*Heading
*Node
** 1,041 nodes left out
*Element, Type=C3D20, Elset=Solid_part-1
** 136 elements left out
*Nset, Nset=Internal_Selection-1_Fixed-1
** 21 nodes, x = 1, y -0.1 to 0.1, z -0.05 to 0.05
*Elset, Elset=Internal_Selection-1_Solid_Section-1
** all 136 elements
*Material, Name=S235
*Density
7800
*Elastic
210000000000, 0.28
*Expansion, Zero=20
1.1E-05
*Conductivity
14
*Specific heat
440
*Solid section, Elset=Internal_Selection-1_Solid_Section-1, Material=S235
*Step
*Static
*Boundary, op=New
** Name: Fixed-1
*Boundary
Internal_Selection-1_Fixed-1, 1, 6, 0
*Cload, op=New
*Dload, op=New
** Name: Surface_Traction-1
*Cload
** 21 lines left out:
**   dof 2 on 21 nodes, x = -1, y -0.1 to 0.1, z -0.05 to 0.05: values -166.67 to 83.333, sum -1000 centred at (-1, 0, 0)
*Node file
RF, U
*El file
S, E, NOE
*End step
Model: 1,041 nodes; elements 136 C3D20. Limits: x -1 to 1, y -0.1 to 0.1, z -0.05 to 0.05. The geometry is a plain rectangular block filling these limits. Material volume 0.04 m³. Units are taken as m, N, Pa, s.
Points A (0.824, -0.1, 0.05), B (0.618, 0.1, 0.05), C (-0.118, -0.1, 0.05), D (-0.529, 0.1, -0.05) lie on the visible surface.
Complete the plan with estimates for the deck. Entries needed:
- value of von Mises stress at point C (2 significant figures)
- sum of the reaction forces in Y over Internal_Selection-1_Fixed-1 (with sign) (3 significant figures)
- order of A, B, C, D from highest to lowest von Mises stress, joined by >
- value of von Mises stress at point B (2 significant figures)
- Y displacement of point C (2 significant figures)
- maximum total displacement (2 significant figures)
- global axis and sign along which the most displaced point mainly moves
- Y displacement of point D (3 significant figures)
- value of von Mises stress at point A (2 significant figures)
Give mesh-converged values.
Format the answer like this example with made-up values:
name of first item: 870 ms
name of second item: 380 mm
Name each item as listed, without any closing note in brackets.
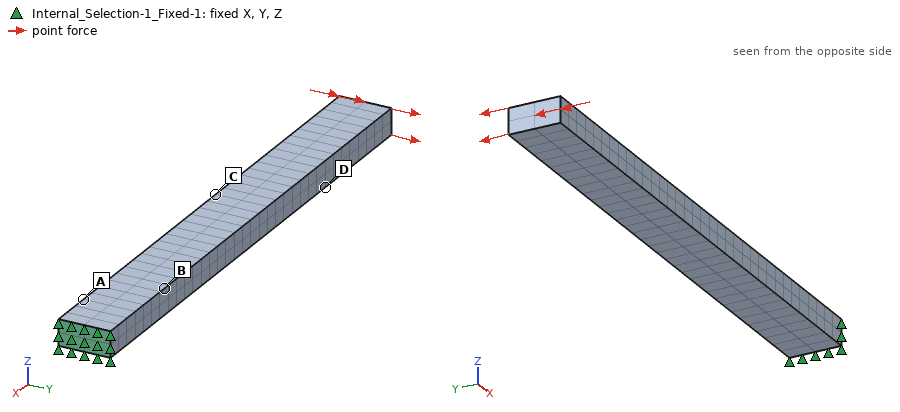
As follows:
value of von Mises stress at point C: 1.3e+06 Pa
sum of the reaction forces in Y over Internal_Selection-1_Fixed-1 (with sign): 1000 N
order of A, B, C, D from highest to lowest von Mises stress, joined by >: A > B > C > D
value of von Mises stress at point B: 2.4e+06 Pa
Y displacement of point C: -7.3e-05 m
maximum total displacement: 1.9e-04 m
global axis and sign along which the most displaced point mainly moves: -Y
Y displacement of point D: -1.25e-04 m
value of von Mises stress at point A: 2.7e+06 Pa
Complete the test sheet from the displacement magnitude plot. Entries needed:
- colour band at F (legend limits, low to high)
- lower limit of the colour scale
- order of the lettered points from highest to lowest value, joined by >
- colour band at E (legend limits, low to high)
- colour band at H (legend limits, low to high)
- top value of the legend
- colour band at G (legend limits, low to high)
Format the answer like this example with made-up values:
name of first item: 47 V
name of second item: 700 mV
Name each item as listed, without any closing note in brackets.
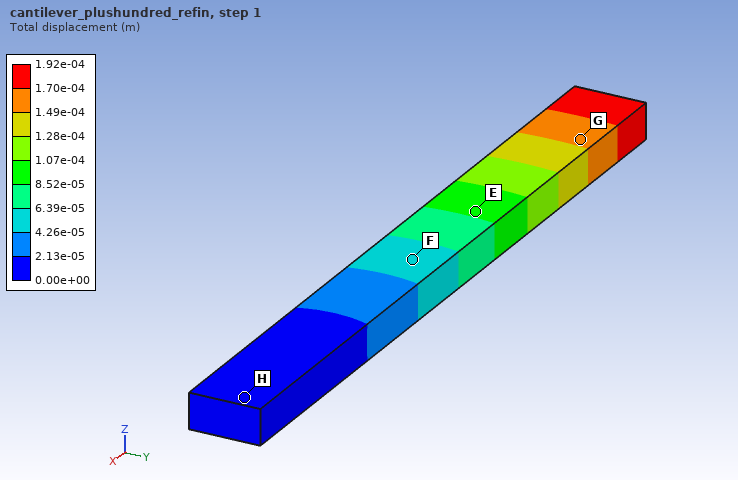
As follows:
colour band at F: 4.26e-05 to 6.39e-05 m
lower limit of the colour scale: 0.00e+00 m
order of the lettered points from highest to lowest value, joined by >: G > E > F > H
colour band at E: 8.52e-05 to 1.07e-04 m
colour band at H: 0.00e+00 to 2.13e-05 m
top value of the legend: 1.92e-04 m
colour band at G: 1.49e-04 to 1.70e-04 m
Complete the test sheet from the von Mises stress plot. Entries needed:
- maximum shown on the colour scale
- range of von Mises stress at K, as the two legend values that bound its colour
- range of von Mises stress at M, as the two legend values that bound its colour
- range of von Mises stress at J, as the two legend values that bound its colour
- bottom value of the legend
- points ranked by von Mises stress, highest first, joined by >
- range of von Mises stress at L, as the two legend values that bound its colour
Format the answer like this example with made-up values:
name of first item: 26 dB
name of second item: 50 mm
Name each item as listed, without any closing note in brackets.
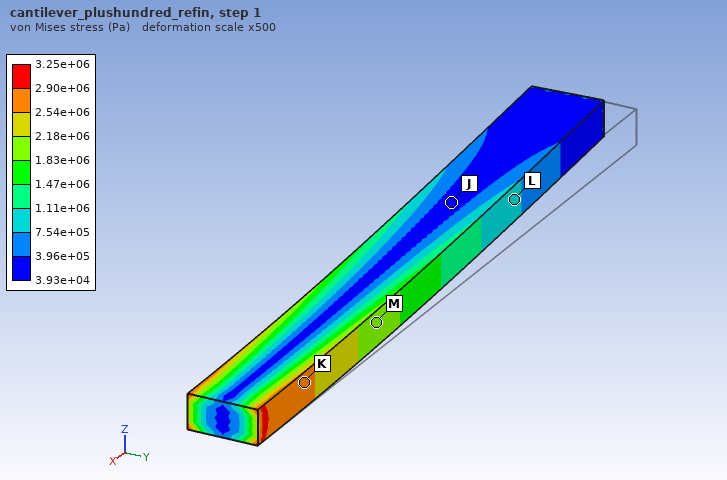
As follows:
maximum shown on the colour scale: 3.25e+06 Pa
range of von Mises stress at K, as the two legend values that bound its colour: 2.54e+06 to 2.90e+06 Pa
range of von Mises stress at M, as the two legend values that bound its colour: 1.83e+06 to 2.18e+06 Pa
range of von Mises stress at J, as the two legend values that bound its colour: 3.93e+04 to 3.96e+05 Pa
bottom value of the legend: 3.93e+04 Pa
points ranked by von Mises stress, highest first, joined by >: K > M > L > J
range of von Mises stress at L, as the two legend values that bound its colour: 7.54e+05 to 1.11e+06 Pa
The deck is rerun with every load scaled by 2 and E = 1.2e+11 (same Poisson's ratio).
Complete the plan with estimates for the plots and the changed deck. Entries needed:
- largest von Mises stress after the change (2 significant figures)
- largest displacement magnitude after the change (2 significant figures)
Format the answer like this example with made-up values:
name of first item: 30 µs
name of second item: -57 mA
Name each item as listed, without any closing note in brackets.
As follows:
largest von Mises stress after the change: 6.5e+06 Pa
largest displacement magnitude after the change: 6.7e-04 m
